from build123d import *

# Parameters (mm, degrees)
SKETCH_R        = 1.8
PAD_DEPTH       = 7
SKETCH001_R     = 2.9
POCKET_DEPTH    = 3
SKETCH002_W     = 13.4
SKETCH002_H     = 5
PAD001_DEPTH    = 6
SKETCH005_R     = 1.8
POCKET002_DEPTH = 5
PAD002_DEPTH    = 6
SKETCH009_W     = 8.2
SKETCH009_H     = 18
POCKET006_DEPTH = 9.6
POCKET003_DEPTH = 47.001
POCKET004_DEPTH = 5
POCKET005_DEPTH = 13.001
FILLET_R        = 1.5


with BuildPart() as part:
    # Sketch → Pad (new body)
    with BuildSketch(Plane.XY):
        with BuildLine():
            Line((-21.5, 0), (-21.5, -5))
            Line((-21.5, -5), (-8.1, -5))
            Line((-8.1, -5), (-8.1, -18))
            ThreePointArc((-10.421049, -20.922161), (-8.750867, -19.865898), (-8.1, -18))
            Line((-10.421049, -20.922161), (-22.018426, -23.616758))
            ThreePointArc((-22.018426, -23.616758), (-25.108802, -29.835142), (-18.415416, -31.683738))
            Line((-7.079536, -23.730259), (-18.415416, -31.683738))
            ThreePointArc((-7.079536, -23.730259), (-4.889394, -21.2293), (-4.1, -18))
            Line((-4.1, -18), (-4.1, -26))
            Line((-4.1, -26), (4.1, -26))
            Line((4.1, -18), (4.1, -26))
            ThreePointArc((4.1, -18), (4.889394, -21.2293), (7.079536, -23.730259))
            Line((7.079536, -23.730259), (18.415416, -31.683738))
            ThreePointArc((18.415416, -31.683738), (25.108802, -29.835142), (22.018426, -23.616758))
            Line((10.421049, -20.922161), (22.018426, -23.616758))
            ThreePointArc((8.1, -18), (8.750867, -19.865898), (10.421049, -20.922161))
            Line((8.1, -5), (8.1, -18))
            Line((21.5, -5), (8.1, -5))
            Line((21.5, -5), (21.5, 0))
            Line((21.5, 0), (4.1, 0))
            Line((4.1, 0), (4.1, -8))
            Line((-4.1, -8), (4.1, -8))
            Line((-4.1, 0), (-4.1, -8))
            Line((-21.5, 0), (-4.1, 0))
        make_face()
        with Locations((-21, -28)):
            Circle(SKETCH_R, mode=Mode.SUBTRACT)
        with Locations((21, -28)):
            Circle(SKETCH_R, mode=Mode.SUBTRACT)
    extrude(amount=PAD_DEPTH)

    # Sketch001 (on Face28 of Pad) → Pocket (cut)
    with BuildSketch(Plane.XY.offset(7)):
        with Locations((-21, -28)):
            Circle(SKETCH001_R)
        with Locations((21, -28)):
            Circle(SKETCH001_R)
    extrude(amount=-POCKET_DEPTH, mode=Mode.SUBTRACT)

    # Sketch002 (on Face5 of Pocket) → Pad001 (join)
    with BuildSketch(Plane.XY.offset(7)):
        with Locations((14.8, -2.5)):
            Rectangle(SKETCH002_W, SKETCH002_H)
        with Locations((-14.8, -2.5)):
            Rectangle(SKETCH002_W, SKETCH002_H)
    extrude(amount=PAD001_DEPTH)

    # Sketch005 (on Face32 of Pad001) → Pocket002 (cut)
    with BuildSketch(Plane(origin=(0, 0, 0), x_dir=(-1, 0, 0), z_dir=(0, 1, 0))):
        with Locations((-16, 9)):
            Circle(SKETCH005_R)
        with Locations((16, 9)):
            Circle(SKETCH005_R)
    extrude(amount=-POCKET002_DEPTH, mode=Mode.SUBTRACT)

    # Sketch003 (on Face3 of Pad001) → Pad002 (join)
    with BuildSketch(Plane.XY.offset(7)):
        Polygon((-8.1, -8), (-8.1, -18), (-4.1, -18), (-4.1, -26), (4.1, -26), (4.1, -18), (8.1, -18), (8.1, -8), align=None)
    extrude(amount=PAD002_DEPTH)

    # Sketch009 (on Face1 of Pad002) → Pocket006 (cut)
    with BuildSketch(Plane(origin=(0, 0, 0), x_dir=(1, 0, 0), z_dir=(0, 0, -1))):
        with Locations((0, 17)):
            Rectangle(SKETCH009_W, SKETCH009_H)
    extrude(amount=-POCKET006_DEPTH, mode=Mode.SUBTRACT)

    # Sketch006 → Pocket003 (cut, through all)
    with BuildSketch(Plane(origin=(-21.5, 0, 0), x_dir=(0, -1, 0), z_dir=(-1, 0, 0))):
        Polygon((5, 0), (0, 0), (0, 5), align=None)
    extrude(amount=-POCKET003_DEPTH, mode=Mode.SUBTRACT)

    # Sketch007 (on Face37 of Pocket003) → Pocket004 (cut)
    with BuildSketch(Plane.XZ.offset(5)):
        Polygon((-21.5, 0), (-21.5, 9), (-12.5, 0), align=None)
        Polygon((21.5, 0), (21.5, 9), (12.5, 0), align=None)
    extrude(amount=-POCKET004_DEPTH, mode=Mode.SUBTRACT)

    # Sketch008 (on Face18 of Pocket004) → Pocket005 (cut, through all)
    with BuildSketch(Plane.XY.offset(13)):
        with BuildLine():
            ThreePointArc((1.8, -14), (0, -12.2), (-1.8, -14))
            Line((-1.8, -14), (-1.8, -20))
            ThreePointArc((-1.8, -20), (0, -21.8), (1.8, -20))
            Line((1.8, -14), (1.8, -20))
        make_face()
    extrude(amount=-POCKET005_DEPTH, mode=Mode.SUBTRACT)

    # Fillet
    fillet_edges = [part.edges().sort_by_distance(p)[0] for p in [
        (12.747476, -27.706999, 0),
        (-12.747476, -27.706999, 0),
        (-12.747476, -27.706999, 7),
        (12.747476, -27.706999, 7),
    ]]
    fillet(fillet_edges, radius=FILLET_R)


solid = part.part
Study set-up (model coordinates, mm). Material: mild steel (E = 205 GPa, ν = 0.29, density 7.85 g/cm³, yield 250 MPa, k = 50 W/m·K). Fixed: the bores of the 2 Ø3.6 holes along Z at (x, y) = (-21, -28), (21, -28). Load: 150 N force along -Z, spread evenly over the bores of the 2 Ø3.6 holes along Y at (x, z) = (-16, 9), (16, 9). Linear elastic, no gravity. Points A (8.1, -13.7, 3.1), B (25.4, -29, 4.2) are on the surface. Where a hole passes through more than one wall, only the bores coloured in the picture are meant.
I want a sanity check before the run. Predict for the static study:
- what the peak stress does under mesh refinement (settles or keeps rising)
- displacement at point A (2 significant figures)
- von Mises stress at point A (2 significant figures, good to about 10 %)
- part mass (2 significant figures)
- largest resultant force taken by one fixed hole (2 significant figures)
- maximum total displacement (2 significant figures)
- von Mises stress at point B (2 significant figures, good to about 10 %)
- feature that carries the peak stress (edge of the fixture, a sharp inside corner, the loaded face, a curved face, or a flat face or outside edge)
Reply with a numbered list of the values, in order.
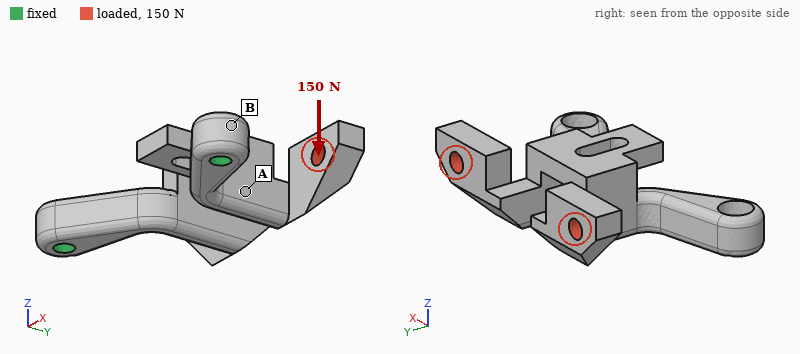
1. keeps rising
2. 22 µm
3. 33 MPa
4. 35 g
5. 80 N
6. 74 µm
7. 14 MPa
8. edge of the fixture
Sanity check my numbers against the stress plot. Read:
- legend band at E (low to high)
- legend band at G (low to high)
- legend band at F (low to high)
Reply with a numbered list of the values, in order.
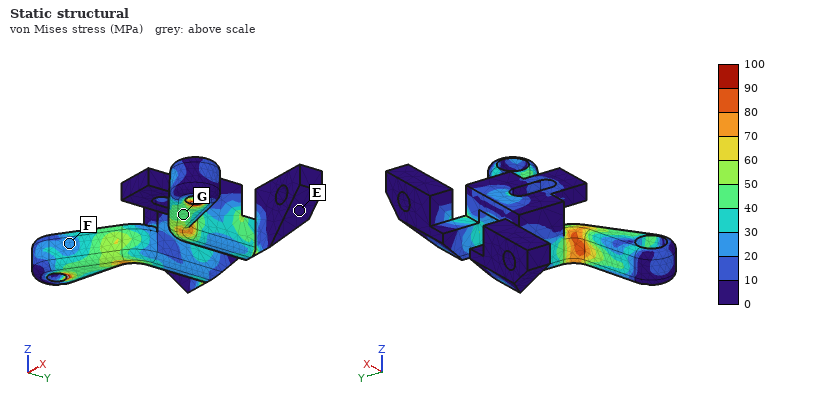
1. 0 to 10 MPa
2. 40 to 50 MPa
3. 20 to 30 MPa
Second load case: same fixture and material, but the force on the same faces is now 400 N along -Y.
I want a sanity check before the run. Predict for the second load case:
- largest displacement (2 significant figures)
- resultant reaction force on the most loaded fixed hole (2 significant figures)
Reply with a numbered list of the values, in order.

1. 98 µm
2. 200 N
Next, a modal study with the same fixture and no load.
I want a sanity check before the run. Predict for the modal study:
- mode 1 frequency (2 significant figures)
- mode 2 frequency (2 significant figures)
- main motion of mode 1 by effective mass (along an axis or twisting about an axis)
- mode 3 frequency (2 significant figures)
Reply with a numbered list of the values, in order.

1. 2300 Hz
2. 3300 Hz
3. along Z
4. 4300 Hz
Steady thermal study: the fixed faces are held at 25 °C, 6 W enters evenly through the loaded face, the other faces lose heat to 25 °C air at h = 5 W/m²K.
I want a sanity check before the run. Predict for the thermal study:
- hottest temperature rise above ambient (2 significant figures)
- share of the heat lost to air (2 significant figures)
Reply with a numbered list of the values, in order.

1. 74 K
2. 10 %
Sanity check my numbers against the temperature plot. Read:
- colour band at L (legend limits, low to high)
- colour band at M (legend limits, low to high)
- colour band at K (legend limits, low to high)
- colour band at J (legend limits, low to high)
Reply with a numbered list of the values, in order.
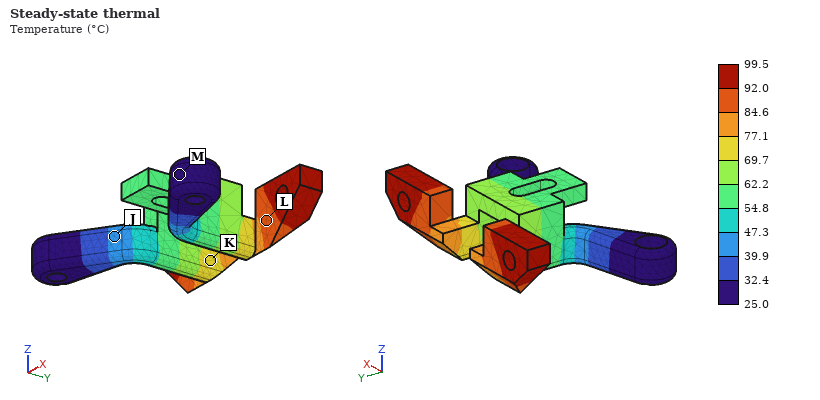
1. 84.6 to 92.0 °C
2. 25.0 to 32.4 °C
3. 69.7 to 77.1 °C
4. 39.9 to 47.3 °C
